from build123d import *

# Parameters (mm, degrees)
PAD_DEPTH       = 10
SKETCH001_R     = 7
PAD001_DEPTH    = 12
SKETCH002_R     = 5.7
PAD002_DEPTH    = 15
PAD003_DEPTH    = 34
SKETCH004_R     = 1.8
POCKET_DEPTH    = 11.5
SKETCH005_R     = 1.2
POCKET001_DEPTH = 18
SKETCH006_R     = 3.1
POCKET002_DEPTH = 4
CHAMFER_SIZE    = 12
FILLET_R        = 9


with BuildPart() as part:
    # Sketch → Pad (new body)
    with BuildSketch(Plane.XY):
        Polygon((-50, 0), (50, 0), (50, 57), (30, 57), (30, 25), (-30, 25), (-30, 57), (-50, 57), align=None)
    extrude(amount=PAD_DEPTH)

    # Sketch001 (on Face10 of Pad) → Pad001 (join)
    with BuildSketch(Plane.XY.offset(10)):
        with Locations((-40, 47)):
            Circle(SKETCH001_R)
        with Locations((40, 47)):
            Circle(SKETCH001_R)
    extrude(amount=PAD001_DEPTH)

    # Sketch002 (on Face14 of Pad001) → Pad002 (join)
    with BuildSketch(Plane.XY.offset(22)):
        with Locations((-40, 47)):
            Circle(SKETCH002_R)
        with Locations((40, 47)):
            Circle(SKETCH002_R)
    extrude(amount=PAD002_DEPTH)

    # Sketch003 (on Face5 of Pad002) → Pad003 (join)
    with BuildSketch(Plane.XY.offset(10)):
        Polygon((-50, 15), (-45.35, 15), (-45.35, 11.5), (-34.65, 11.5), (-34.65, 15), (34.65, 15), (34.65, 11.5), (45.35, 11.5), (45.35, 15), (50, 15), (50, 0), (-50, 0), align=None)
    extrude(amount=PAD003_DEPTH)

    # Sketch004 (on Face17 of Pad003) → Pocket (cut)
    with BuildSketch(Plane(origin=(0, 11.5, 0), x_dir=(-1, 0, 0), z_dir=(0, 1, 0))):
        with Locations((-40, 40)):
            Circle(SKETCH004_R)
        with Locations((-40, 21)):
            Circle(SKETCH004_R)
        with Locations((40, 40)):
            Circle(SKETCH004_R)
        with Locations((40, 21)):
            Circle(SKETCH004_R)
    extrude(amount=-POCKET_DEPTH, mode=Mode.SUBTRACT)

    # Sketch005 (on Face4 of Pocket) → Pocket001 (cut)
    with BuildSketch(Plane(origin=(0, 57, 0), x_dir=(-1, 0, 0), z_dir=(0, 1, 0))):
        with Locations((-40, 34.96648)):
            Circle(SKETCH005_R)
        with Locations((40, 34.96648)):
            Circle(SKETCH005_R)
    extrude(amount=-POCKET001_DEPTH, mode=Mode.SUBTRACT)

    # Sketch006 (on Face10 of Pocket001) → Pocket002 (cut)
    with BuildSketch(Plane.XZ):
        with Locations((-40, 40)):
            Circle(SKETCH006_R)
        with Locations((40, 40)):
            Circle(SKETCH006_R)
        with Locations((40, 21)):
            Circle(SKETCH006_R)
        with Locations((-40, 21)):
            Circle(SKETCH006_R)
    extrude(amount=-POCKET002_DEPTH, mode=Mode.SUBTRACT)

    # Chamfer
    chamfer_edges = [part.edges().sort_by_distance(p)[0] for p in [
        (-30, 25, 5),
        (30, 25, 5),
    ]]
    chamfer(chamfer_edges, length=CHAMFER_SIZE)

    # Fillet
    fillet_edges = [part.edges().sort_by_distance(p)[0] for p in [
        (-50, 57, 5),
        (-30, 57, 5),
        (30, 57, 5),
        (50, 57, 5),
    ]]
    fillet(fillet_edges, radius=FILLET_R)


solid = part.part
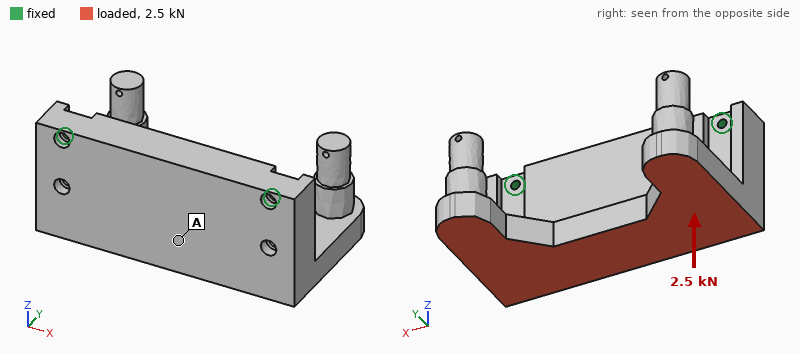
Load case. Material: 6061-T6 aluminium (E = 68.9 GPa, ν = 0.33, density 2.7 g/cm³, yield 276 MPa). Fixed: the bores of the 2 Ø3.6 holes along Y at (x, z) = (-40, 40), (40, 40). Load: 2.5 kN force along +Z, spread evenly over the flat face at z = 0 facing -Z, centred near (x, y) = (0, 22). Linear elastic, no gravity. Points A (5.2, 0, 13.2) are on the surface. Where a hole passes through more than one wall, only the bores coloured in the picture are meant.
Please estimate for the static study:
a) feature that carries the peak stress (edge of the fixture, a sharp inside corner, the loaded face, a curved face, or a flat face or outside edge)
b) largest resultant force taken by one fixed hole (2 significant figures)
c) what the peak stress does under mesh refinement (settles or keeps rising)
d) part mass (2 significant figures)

edge of the fixture
1.3 kN
keeps rising
250 g
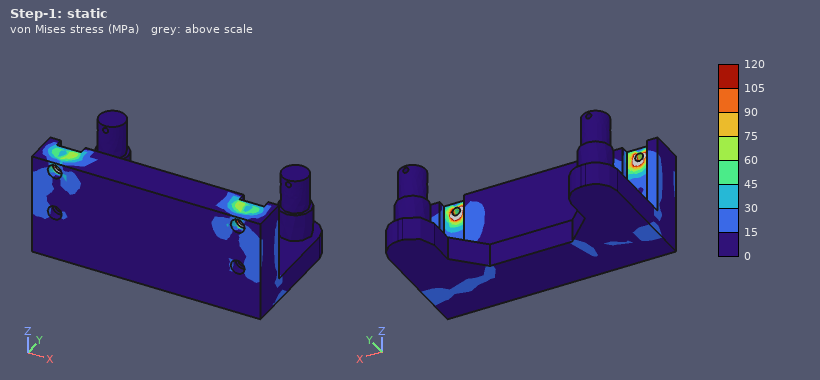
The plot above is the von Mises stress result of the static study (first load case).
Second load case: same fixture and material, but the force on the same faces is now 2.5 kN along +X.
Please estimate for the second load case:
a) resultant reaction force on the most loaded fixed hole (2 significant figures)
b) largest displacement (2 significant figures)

1.8 kN
37 µm
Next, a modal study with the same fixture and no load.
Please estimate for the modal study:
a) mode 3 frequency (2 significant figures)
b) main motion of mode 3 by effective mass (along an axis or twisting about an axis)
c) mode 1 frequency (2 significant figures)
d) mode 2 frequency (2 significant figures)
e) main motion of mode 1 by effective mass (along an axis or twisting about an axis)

3100 Hz
along Y
1200 Hz
2500 Hz
along Y
